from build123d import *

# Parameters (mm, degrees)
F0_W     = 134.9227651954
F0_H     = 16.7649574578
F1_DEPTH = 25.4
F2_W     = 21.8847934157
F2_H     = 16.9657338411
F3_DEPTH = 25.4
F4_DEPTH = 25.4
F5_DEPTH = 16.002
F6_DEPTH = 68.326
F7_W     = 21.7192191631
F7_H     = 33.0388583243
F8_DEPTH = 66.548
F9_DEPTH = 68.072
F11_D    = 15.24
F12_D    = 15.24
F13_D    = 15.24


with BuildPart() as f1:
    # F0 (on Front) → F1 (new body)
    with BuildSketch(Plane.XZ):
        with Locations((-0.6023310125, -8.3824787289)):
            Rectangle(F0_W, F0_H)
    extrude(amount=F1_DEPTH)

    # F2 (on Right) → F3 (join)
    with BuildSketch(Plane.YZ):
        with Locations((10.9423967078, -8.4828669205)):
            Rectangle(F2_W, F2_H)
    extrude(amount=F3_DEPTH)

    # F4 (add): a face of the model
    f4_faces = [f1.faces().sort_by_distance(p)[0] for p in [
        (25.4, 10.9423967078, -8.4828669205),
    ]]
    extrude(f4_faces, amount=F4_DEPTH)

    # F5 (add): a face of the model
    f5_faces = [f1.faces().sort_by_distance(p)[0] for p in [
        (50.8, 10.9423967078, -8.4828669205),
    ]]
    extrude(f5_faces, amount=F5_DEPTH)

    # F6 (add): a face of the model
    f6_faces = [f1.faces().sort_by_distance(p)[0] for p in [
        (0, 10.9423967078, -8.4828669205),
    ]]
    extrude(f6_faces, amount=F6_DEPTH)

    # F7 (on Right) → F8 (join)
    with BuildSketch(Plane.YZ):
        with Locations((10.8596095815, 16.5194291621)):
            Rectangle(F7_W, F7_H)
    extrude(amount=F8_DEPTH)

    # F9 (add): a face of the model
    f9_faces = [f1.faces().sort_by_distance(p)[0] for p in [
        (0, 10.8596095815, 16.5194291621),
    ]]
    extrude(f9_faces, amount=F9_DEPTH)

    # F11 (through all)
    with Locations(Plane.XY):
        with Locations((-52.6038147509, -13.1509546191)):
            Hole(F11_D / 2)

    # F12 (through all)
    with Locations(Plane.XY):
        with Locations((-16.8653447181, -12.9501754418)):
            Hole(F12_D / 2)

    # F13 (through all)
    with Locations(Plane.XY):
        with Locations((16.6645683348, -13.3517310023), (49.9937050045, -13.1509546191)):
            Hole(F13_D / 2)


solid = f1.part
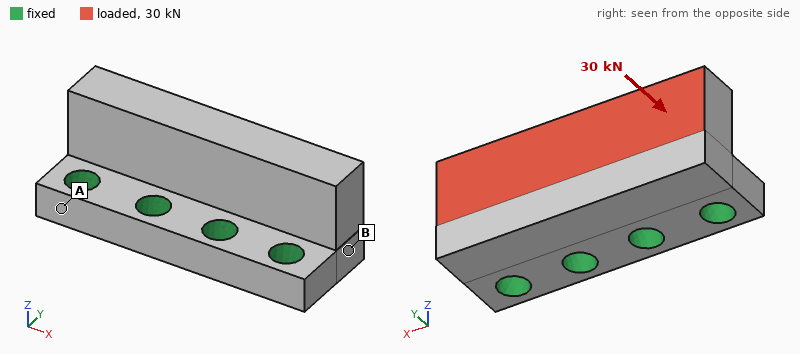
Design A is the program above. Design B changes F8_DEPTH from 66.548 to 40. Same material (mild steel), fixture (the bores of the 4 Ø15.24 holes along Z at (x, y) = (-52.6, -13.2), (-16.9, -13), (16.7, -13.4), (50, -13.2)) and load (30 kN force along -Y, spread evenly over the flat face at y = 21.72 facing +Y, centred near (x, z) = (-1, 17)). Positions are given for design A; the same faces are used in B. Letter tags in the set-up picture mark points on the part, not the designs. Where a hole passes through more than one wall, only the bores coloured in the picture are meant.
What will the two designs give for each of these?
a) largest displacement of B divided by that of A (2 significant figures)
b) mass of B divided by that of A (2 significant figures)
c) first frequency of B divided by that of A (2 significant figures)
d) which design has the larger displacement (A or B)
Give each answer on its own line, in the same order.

1.2
0.90
1.0
B
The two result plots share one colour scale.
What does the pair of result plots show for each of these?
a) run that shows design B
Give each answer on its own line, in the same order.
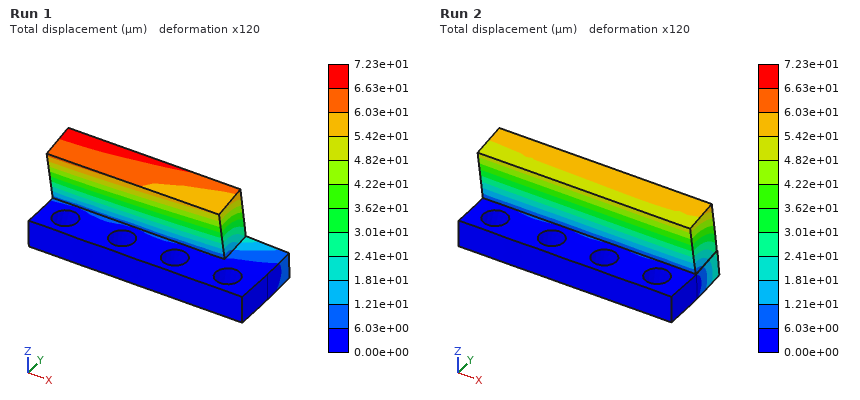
Run 1
